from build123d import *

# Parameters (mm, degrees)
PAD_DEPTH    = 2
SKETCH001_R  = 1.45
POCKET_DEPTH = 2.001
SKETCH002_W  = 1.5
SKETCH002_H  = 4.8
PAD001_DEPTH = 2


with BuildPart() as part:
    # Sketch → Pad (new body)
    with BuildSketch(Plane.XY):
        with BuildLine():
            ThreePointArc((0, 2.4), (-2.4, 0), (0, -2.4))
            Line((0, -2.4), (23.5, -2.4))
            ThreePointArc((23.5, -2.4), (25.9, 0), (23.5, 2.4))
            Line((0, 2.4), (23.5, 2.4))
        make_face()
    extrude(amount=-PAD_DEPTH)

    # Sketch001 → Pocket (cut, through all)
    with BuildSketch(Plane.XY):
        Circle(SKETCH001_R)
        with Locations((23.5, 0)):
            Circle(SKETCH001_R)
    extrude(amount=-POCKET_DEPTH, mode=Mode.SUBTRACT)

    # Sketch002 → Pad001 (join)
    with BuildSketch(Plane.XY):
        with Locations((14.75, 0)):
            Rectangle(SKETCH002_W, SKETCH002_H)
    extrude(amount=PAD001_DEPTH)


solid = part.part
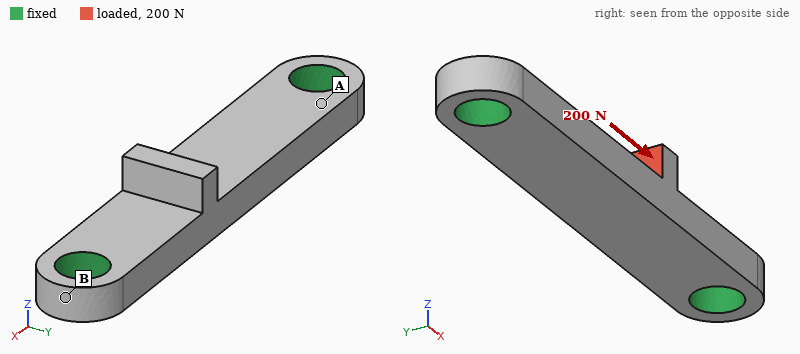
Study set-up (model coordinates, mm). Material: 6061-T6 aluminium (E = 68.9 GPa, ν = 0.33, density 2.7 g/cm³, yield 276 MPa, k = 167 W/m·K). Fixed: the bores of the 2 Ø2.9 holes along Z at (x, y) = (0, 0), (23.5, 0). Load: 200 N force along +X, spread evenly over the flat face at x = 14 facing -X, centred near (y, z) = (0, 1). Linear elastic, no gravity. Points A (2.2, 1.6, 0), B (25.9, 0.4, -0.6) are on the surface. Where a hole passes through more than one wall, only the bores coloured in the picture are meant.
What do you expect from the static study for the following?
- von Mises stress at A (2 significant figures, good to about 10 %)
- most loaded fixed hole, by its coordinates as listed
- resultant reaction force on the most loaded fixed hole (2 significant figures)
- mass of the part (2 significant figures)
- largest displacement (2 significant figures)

20 MPa
(23.5, 0)
130 N
0.67 g
17 µm
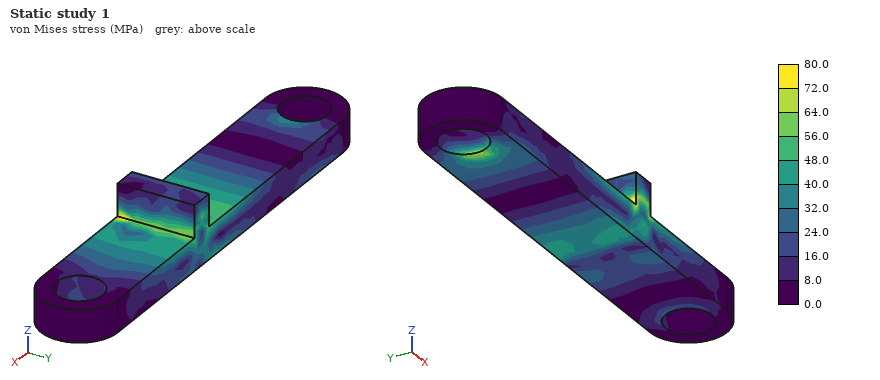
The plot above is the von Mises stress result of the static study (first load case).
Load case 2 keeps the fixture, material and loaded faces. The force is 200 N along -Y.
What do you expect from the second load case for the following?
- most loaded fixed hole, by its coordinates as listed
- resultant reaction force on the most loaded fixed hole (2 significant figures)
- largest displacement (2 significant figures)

(23.5, 0)
130 N
41 µm
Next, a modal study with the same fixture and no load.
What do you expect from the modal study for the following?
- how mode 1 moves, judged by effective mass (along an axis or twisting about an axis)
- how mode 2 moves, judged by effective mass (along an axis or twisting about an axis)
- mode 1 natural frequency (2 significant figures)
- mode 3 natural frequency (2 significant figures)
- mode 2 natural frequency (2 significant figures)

along Z
along Y
21 kHz
45 kHz
35 kHz
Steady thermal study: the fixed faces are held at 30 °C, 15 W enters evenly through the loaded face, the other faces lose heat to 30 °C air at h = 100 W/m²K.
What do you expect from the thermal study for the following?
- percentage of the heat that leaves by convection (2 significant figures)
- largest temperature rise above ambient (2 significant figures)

4.9 %
64 K
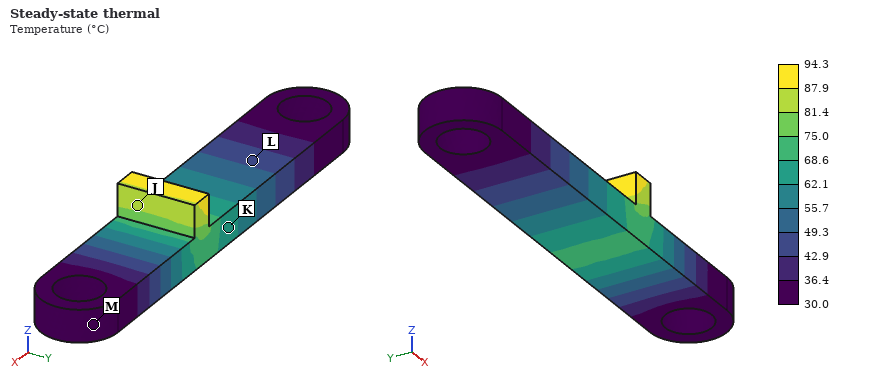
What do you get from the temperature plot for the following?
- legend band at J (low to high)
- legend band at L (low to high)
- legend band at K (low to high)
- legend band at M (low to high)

81.4 to 87.9 °C
42.9 to 49.3 °C
62.1 to 68.6 °C
30.0 to 36.4 °C
